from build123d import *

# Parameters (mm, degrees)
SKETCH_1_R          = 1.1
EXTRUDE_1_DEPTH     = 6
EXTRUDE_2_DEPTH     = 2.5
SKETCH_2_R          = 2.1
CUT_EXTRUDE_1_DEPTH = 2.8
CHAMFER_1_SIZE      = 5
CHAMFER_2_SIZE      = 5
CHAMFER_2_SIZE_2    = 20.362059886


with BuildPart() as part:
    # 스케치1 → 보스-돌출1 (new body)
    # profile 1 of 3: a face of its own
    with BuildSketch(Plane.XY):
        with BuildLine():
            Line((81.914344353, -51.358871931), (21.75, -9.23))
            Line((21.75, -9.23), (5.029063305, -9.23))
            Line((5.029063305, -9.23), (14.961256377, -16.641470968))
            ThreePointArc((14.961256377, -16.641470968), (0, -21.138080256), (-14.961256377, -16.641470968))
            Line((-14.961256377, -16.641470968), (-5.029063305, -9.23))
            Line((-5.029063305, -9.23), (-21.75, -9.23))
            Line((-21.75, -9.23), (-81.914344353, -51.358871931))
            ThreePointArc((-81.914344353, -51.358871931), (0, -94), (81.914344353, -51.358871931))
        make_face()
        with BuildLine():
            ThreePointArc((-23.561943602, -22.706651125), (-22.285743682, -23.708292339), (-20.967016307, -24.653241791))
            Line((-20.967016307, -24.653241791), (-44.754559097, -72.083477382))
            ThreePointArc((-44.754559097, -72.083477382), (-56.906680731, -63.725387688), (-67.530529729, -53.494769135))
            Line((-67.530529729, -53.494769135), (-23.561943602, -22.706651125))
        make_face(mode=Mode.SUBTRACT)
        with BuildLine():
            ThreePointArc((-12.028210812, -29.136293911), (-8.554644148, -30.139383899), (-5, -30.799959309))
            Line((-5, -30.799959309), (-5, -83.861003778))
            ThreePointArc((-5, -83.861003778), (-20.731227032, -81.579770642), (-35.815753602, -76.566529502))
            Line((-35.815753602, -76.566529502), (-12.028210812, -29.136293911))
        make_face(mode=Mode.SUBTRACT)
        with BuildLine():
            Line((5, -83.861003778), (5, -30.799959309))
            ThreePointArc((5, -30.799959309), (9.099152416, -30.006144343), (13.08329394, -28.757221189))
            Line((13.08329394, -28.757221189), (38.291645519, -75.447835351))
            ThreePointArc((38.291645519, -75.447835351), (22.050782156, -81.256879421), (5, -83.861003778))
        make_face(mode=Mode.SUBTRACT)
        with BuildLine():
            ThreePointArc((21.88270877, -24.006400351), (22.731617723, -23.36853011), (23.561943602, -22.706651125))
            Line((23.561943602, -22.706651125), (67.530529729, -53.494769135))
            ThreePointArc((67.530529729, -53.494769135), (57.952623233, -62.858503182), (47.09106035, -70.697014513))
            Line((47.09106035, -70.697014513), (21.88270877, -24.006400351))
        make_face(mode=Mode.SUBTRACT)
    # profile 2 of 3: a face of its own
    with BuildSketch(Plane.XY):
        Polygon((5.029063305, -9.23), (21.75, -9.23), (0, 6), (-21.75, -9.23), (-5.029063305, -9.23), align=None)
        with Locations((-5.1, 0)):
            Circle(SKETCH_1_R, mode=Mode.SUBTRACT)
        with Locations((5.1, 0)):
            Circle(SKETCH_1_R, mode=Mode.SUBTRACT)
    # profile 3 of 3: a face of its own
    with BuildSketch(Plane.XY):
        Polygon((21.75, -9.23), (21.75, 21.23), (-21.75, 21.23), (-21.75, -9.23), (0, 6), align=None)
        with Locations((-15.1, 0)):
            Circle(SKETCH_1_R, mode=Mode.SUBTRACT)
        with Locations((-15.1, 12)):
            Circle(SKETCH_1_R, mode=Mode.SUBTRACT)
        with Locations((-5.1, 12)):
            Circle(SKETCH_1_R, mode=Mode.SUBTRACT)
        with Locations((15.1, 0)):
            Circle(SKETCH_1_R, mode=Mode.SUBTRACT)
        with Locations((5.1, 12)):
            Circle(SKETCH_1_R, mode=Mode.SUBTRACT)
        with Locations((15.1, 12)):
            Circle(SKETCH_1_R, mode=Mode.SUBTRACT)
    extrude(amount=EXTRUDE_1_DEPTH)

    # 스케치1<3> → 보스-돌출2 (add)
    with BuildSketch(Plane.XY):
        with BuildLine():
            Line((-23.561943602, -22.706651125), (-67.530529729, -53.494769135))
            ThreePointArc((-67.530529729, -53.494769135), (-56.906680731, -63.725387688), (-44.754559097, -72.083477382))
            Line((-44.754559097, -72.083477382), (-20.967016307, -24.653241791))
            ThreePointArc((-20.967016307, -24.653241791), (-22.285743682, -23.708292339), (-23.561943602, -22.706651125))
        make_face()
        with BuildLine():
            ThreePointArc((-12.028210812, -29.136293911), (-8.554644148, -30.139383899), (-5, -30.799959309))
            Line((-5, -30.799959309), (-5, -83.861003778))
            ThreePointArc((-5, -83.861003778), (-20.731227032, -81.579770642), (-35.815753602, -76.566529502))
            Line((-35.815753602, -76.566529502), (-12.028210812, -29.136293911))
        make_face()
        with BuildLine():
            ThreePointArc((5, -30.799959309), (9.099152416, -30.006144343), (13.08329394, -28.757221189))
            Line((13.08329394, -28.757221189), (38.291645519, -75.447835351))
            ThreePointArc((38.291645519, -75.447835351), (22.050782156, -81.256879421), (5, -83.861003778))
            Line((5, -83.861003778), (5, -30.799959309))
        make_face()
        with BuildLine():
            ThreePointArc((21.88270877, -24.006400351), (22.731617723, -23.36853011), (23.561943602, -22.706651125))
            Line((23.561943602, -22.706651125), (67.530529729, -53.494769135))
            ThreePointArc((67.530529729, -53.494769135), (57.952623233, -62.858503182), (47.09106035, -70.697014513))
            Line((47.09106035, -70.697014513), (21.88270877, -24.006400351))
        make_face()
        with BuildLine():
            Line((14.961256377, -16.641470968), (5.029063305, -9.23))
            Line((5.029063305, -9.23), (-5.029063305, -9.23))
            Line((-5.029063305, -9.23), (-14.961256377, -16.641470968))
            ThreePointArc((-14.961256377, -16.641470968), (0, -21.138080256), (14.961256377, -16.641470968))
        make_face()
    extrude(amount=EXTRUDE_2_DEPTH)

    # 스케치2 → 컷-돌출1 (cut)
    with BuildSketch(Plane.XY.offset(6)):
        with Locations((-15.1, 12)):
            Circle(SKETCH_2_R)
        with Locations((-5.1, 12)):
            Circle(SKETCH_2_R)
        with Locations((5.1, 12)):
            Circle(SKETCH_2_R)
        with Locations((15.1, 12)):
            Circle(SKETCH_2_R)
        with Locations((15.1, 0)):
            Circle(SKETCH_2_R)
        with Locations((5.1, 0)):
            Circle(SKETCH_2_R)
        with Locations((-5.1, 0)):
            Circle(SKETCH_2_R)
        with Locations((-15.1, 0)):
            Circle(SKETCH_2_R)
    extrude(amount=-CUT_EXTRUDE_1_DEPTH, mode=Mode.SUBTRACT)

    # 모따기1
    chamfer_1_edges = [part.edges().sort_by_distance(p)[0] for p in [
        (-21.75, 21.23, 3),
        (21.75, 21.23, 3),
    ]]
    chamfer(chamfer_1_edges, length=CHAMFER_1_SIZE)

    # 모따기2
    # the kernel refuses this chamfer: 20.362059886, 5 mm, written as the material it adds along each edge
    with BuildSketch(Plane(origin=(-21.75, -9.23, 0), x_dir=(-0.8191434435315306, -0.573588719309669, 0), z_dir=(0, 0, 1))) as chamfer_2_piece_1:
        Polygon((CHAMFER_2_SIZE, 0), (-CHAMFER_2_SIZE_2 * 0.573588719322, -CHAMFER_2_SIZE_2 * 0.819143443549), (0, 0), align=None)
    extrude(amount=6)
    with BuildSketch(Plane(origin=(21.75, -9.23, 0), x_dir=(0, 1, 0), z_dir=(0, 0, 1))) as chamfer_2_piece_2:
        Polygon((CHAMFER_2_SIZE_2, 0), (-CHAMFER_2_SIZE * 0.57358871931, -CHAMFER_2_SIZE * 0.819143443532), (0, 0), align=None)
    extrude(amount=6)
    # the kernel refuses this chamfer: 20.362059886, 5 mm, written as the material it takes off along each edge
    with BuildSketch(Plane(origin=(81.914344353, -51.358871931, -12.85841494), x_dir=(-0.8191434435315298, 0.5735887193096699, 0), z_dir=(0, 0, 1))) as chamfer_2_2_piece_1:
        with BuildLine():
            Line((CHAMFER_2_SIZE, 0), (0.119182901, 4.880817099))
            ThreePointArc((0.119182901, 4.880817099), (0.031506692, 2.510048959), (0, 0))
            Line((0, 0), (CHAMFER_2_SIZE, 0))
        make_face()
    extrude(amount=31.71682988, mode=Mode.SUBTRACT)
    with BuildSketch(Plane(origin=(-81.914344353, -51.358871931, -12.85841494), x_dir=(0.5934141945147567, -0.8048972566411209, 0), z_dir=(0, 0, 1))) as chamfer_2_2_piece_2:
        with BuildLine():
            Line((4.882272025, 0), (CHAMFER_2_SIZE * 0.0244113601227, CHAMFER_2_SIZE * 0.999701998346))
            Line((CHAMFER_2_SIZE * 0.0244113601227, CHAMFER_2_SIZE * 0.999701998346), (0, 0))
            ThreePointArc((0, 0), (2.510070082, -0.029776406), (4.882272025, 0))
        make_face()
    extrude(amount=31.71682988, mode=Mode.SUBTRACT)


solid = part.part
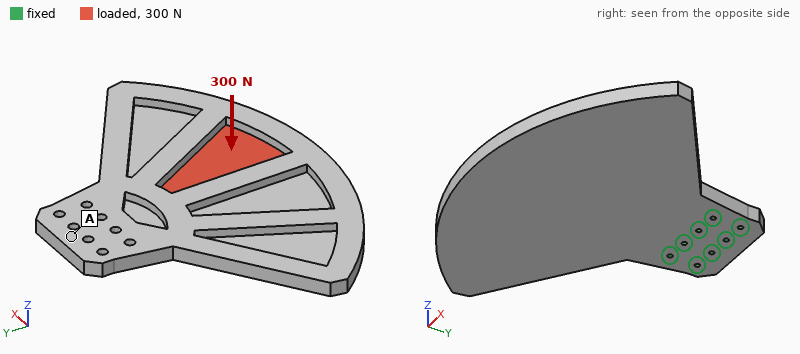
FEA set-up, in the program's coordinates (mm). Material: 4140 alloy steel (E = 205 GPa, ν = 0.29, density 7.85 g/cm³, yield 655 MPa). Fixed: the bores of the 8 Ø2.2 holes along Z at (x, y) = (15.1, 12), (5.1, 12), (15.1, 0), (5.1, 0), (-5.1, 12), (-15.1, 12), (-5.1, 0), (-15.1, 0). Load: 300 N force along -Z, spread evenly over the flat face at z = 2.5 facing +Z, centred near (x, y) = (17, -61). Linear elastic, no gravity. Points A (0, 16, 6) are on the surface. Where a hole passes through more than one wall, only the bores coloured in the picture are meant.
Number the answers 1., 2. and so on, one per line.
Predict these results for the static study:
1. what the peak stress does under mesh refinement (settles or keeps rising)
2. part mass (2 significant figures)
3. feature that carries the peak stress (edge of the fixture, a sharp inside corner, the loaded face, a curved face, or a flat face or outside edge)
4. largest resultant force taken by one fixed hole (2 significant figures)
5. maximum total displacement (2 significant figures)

1. keeps rising
2. 390 g
3. edge of the fixture
4. 640 N
5. 0.32 mm
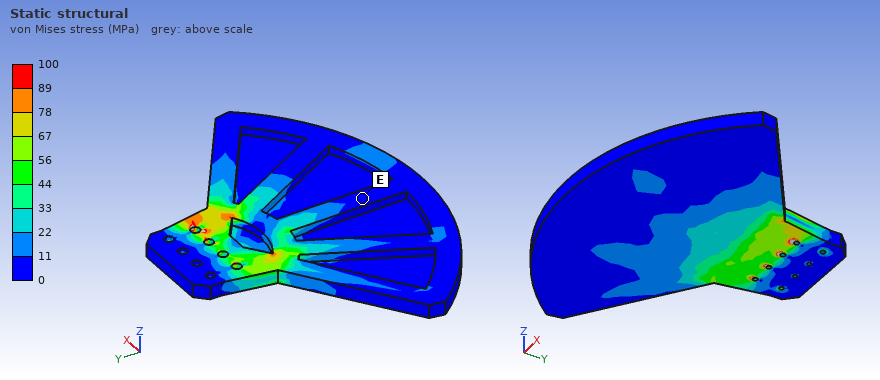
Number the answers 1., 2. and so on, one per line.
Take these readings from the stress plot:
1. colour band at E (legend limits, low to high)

1. 0 to 11 MPa
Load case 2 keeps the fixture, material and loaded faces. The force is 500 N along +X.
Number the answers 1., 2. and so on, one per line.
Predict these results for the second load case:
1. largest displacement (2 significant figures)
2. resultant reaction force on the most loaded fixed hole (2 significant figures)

1. 13 µm
2. 600 N
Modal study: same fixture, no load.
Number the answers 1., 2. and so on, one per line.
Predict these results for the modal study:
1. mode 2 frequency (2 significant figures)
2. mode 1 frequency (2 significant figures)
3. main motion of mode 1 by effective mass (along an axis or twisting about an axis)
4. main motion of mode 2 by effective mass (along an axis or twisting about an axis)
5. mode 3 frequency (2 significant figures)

1. 590 Hz
2. 390 Hz
3. along Z
4. twisting about Y
5. 1300 Hz
